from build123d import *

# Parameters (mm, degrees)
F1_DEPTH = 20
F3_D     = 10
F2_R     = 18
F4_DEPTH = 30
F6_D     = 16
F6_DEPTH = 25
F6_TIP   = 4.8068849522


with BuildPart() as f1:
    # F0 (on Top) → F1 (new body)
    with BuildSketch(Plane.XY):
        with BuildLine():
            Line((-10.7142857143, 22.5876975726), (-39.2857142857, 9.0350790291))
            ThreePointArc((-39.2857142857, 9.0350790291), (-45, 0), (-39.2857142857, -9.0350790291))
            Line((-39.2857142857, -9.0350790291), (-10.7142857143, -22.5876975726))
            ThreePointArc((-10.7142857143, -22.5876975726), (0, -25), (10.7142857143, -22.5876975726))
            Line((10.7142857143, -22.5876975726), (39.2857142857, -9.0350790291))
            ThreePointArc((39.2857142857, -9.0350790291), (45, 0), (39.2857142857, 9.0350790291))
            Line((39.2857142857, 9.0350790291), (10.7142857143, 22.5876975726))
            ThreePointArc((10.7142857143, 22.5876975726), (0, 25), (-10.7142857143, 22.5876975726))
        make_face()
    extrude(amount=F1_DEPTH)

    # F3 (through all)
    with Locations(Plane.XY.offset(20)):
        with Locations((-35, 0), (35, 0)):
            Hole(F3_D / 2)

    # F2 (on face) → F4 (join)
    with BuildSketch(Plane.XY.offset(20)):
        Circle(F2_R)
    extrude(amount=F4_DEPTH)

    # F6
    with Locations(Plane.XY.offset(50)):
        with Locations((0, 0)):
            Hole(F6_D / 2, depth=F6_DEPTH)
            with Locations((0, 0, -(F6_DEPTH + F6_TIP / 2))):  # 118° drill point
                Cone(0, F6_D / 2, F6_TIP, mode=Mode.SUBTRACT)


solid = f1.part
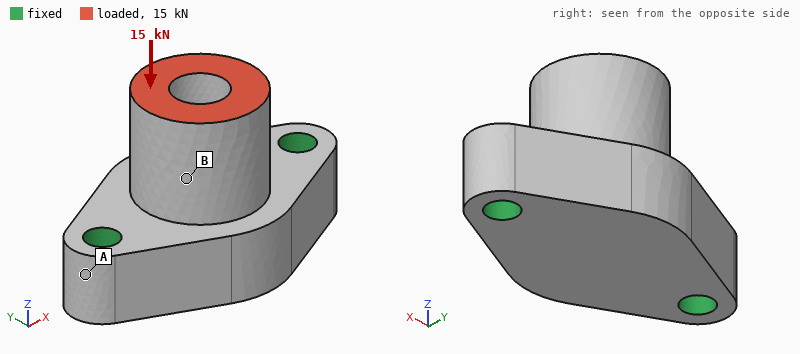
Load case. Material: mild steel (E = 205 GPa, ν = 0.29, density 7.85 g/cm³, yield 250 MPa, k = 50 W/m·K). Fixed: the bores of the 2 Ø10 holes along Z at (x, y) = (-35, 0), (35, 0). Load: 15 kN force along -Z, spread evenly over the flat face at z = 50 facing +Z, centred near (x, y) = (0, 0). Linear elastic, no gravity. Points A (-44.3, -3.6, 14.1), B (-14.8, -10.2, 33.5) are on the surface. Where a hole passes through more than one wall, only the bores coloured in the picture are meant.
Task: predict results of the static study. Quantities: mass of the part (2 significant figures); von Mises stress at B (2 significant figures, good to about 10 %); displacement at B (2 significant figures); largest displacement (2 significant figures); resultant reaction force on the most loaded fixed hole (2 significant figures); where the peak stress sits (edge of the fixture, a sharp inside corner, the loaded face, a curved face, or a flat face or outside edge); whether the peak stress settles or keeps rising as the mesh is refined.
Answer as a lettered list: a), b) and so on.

a) 640 g
b) 19 MPa
c) 7.3 µm
d) 8.8 µm
e) 7.6 kN
f) edge of the fixture
g) keeps rising
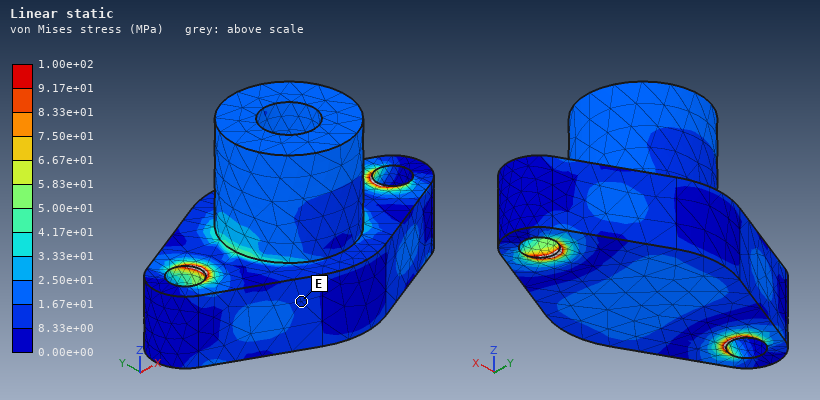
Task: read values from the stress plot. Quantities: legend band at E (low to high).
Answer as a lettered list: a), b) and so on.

a) 8.33e+00 to 1.67e+01 MPa
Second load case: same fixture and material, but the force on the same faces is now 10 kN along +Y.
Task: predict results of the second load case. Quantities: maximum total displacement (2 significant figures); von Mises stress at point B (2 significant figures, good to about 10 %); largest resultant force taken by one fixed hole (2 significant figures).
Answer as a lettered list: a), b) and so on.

a) 65 µm
b) 34 MPa
c) 5.0 kN
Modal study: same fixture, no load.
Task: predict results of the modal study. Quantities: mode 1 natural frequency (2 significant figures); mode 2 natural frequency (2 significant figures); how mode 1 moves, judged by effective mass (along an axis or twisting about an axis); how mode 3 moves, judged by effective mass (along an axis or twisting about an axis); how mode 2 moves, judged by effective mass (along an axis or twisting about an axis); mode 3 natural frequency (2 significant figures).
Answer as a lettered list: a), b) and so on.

a) 6200 Hz
b) 11 kHz
c) along Y
d) along X
e) along Z
f) 12 kHz
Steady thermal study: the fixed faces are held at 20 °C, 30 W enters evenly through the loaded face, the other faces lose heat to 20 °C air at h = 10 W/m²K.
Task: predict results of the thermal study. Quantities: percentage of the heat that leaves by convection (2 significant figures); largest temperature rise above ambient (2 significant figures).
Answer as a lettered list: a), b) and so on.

a) 5.4 %
b) 34 K
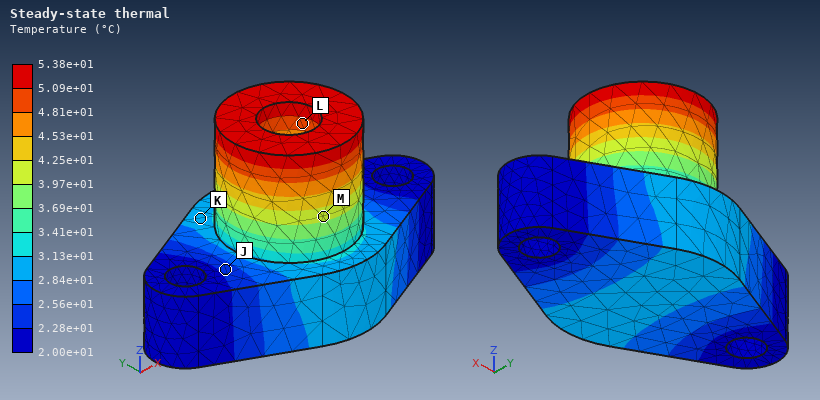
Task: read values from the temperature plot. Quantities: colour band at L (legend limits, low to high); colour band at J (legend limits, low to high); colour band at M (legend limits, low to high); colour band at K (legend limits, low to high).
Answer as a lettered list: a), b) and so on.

a) 4.81e+01 to 5.09e+01 °C
b) 2.28e+01 to 2.56e+01 °C
c) 3.97e+01 to 4.25e+01 °C
d) 2.84e+01 to 3.13e+01 °C
